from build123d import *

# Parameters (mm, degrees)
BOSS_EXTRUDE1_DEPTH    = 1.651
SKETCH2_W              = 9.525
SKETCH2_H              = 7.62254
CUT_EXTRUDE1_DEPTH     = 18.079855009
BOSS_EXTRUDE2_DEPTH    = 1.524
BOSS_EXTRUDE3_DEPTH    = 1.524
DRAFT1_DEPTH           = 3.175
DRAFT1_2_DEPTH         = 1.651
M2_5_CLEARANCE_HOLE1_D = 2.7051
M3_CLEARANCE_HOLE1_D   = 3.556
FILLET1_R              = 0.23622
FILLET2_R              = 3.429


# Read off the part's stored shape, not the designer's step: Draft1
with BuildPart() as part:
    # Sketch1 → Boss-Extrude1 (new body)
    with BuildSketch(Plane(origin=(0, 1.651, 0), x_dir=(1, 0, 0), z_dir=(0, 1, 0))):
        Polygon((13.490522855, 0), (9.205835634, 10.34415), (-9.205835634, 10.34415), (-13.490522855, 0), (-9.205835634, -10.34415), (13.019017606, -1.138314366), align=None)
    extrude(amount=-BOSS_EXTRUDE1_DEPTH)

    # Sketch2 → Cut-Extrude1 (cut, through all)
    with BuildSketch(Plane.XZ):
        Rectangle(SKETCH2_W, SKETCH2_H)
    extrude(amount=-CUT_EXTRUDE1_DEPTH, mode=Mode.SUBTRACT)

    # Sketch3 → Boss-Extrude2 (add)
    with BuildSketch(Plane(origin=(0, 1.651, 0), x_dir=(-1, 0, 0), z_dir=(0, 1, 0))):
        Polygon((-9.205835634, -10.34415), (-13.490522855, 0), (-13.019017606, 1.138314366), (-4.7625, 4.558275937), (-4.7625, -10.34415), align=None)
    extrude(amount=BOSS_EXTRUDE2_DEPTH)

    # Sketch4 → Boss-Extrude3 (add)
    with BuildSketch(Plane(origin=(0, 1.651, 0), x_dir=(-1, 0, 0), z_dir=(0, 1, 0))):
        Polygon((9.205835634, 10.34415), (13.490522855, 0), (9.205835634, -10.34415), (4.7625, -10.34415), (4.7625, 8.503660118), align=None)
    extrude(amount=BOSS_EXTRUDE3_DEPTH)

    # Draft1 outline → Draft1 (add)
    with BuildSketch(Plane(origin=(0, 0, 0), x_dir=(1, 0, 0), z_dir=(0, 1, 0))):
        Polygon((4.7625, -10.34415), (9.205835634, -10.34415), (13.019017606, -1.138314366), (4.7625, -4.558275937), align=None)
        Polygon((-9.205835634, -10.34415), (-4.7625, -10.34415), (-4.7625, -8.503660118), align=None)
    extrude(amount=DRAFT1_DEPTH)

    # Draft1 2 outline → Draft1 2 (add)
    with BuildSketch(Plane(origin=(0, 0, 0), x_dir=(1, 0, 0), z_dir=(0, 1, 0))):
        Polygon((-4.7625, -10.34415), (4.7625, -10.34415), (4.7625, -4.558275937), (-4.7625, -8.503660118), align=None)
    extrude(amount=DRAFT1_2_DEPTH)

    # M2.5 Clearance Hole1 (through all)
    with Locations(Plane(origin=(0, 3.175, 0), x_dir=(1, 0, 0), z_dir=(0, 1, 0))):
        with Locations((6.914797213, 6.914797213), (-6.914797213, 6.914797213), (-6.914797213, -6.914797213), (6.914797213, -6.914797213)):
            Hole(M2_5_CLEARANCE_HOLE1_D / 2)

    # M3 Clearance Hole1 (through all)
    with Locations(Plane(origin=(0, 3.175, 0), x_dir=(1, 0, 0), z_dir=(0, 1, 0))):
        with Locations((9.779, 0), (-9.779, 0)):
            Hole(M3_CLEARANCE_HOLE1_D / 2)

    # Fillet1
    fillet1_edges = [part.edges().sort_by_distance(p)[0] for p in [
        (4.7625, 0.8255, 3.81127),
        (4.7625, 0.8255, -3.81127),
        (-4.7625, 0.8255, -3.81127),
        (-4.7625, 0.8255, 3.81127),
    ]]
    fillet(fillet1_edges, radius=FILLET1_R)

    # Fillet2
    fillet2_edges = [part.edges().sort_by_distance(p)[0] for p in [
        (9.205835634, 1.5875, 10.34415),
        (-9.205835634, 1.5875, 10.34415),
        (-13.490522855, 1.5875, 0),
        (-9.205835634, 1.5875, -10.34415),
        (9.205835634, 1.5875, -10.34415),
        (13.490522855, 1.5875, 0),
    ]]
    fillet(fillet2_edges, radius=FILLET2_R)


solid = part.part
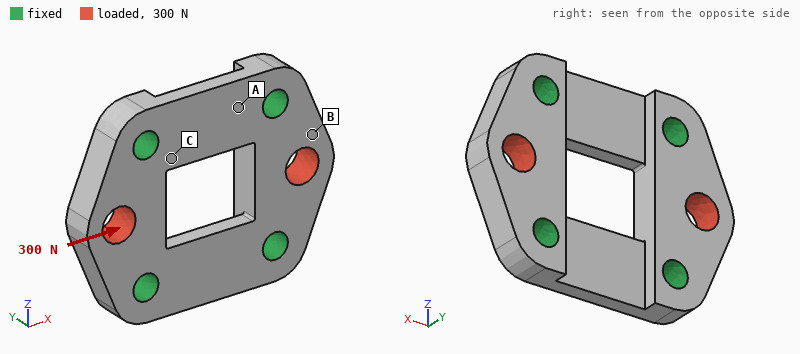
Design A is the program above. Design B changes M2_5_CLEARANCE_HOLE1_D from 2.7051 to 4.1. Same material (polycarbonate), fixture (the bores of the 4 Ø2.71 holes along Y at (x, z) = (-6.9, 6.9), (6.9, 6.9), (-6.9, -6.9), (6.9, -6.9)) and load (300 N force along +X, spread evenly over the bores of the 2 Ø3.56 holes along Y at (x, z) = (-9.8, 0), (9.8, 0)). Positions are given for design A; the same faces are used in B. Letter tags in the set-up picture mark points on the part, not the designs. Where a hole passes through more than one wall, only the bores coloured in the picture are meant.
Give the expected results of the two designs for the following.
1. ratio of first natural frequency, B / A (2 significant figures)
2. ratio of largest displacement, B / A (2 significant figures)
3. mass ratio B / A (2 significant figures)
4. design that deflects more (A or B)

1.2
0.87
0.90
A
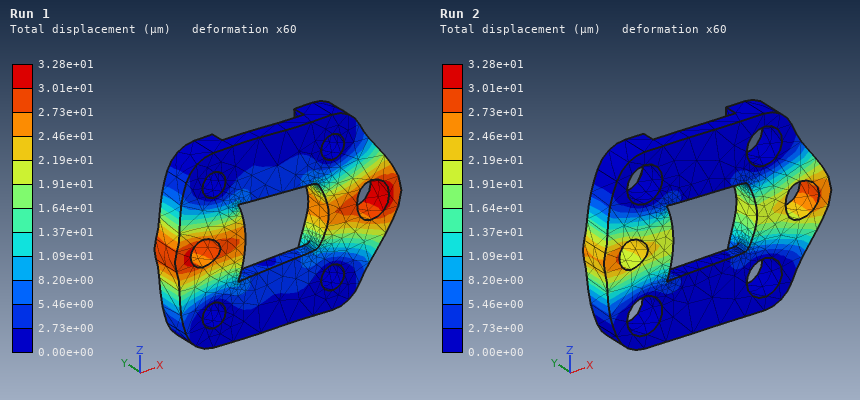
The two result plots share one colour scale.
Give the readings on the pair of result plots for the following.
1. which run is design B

Run 2
